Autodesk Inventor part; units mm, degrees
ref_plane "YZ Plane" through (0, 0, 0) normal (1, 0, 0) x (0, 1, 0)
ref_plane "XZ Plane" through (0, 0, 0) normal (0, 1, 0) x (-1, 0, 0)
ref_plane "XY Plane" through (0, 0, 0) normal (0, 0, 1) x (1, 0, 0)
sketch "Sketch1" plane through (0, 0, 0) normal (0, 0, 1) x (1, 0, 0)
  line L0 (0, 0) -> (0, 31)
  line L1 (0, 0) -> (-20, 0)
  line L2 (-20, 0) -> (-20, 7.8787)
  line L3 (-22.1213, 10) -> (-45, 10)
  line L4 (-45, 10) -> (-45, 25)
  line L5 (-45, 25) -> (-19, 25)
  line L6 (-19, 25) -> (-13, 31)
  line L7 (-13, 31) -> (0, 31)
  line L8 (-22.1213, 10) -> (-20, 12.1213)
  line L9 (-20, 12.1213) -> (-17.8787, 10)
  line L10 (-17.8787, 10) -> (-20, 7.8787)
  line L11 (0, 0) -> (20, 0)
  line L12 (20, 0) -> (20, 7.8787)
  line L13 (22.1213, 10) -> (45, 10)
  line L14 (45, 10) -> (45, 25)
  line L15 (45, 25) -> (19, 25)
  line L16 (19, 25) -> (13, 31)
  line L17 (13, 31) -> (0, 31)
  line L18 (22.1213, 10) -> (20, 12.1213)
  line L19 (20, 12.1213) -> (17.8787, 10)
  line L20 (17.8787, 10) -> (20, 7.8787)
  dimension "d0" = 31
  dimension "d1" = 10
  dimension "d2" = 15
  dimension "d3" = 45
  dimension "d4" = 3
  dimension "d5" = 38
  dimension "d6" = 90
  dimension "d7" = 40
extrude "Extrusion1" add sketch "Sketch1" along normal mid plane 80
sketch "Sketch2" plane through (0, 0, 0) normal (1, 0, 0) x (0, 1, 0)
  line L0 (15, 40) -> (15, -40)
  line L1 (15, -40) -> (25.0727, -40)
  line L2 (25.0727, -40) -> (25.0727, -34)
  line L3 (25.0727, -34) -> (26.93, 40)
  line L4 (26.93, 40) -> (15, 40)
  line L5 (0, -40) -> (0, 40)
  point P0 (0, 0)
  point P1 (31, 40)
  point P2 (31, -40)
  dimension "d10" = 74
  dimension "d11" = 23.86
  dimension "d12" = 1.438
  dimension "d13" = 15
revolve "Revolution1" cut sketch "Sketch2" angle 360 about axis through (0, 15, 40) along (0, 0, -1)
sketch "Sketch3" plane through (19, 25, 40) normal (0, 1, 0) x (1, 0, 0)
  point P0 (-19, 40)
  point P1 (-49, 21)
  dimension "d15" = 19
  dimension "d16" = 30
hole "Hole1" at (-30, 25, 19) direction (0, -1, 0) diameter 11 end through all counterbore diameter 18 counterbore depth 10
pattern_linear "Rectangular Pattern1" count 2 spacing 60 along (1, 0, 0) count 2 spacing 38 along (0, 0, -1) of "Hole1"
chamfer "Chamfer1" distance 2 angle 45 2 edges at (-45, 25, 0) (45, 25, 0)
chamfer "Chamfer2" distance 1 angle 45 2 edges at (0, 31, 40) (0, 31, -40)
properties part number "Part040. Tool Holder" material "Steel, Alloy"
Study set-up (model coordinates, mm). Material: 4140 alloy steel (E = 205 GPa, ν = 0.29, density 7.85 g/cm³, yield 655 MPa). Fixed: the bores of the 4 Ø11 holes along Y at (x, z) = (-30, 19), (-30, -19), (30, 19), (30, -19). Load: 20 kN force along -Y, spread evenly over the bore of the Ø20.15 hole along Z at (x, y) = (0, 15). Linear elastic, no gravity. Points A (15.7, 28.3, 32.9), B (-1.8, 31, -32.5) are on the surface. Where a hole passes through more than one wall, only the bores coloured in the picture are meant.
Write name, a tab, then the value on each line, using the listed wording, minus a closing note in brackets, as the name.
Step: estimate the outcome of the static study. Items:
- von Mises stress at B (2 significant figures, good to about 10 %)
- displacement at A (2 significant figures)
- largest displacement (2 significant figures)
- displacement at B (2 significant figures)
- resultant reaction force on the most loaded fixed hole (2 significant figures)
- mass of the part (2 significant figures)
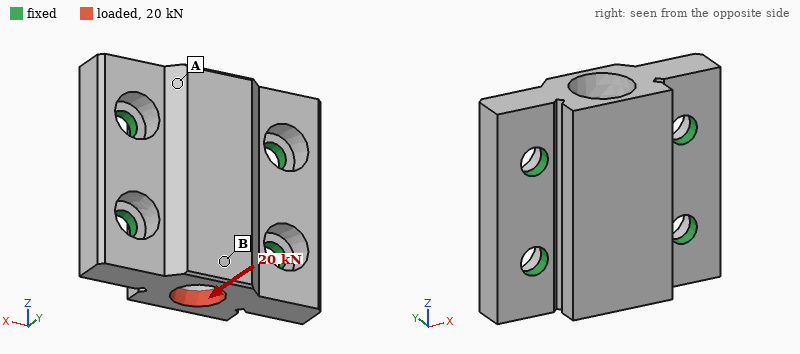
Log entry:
von Mises stress at B	100 MPa
displacement at A	7.8 µm
largest displacement	48 µm
displacement at B	34 µm
resultant reaction force on the most loaded fixed hole	14 kN
mass of the part	880 g
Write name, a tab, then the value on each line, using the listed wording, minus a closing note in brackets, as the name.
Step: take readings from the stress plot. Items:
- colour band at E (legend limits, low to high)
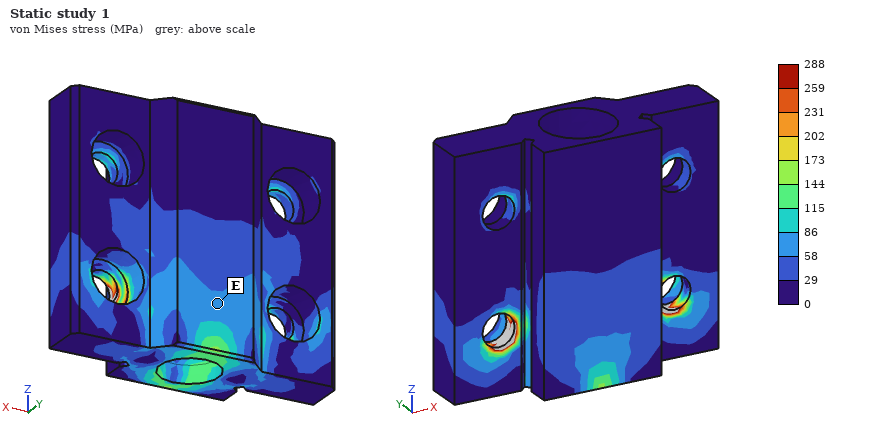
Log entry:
colour band at E	58 to 86 MPa
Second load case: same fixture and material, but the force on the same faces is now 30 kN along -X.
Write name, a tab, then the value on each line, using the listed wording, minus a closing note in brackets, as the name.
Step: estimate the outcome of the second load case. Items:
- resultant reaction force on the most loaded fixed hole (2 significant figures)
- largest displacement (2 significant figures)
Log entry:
resultant reaction force on the most loaded fixed hole	15 kN
largest displacement	20 µm
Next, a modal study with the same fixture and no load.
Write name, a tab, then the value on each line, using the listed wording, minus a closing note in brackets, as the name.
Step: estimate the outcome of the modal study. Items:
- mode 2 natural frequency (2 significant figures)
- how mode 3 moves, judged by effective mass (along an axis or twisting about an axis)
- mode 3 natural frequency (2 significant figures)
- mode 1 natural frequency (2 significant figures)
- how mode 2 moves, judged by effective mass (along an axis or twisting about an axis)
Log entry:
mode 2 natural frequency	12 kHz
how mode 3 moves, judged by effective mass	along X
mode 3 natural frequency	14 kHz
mode 1 natural frequency	9800 Hz
how mode 2 moves, judged by effective mass	along Y
